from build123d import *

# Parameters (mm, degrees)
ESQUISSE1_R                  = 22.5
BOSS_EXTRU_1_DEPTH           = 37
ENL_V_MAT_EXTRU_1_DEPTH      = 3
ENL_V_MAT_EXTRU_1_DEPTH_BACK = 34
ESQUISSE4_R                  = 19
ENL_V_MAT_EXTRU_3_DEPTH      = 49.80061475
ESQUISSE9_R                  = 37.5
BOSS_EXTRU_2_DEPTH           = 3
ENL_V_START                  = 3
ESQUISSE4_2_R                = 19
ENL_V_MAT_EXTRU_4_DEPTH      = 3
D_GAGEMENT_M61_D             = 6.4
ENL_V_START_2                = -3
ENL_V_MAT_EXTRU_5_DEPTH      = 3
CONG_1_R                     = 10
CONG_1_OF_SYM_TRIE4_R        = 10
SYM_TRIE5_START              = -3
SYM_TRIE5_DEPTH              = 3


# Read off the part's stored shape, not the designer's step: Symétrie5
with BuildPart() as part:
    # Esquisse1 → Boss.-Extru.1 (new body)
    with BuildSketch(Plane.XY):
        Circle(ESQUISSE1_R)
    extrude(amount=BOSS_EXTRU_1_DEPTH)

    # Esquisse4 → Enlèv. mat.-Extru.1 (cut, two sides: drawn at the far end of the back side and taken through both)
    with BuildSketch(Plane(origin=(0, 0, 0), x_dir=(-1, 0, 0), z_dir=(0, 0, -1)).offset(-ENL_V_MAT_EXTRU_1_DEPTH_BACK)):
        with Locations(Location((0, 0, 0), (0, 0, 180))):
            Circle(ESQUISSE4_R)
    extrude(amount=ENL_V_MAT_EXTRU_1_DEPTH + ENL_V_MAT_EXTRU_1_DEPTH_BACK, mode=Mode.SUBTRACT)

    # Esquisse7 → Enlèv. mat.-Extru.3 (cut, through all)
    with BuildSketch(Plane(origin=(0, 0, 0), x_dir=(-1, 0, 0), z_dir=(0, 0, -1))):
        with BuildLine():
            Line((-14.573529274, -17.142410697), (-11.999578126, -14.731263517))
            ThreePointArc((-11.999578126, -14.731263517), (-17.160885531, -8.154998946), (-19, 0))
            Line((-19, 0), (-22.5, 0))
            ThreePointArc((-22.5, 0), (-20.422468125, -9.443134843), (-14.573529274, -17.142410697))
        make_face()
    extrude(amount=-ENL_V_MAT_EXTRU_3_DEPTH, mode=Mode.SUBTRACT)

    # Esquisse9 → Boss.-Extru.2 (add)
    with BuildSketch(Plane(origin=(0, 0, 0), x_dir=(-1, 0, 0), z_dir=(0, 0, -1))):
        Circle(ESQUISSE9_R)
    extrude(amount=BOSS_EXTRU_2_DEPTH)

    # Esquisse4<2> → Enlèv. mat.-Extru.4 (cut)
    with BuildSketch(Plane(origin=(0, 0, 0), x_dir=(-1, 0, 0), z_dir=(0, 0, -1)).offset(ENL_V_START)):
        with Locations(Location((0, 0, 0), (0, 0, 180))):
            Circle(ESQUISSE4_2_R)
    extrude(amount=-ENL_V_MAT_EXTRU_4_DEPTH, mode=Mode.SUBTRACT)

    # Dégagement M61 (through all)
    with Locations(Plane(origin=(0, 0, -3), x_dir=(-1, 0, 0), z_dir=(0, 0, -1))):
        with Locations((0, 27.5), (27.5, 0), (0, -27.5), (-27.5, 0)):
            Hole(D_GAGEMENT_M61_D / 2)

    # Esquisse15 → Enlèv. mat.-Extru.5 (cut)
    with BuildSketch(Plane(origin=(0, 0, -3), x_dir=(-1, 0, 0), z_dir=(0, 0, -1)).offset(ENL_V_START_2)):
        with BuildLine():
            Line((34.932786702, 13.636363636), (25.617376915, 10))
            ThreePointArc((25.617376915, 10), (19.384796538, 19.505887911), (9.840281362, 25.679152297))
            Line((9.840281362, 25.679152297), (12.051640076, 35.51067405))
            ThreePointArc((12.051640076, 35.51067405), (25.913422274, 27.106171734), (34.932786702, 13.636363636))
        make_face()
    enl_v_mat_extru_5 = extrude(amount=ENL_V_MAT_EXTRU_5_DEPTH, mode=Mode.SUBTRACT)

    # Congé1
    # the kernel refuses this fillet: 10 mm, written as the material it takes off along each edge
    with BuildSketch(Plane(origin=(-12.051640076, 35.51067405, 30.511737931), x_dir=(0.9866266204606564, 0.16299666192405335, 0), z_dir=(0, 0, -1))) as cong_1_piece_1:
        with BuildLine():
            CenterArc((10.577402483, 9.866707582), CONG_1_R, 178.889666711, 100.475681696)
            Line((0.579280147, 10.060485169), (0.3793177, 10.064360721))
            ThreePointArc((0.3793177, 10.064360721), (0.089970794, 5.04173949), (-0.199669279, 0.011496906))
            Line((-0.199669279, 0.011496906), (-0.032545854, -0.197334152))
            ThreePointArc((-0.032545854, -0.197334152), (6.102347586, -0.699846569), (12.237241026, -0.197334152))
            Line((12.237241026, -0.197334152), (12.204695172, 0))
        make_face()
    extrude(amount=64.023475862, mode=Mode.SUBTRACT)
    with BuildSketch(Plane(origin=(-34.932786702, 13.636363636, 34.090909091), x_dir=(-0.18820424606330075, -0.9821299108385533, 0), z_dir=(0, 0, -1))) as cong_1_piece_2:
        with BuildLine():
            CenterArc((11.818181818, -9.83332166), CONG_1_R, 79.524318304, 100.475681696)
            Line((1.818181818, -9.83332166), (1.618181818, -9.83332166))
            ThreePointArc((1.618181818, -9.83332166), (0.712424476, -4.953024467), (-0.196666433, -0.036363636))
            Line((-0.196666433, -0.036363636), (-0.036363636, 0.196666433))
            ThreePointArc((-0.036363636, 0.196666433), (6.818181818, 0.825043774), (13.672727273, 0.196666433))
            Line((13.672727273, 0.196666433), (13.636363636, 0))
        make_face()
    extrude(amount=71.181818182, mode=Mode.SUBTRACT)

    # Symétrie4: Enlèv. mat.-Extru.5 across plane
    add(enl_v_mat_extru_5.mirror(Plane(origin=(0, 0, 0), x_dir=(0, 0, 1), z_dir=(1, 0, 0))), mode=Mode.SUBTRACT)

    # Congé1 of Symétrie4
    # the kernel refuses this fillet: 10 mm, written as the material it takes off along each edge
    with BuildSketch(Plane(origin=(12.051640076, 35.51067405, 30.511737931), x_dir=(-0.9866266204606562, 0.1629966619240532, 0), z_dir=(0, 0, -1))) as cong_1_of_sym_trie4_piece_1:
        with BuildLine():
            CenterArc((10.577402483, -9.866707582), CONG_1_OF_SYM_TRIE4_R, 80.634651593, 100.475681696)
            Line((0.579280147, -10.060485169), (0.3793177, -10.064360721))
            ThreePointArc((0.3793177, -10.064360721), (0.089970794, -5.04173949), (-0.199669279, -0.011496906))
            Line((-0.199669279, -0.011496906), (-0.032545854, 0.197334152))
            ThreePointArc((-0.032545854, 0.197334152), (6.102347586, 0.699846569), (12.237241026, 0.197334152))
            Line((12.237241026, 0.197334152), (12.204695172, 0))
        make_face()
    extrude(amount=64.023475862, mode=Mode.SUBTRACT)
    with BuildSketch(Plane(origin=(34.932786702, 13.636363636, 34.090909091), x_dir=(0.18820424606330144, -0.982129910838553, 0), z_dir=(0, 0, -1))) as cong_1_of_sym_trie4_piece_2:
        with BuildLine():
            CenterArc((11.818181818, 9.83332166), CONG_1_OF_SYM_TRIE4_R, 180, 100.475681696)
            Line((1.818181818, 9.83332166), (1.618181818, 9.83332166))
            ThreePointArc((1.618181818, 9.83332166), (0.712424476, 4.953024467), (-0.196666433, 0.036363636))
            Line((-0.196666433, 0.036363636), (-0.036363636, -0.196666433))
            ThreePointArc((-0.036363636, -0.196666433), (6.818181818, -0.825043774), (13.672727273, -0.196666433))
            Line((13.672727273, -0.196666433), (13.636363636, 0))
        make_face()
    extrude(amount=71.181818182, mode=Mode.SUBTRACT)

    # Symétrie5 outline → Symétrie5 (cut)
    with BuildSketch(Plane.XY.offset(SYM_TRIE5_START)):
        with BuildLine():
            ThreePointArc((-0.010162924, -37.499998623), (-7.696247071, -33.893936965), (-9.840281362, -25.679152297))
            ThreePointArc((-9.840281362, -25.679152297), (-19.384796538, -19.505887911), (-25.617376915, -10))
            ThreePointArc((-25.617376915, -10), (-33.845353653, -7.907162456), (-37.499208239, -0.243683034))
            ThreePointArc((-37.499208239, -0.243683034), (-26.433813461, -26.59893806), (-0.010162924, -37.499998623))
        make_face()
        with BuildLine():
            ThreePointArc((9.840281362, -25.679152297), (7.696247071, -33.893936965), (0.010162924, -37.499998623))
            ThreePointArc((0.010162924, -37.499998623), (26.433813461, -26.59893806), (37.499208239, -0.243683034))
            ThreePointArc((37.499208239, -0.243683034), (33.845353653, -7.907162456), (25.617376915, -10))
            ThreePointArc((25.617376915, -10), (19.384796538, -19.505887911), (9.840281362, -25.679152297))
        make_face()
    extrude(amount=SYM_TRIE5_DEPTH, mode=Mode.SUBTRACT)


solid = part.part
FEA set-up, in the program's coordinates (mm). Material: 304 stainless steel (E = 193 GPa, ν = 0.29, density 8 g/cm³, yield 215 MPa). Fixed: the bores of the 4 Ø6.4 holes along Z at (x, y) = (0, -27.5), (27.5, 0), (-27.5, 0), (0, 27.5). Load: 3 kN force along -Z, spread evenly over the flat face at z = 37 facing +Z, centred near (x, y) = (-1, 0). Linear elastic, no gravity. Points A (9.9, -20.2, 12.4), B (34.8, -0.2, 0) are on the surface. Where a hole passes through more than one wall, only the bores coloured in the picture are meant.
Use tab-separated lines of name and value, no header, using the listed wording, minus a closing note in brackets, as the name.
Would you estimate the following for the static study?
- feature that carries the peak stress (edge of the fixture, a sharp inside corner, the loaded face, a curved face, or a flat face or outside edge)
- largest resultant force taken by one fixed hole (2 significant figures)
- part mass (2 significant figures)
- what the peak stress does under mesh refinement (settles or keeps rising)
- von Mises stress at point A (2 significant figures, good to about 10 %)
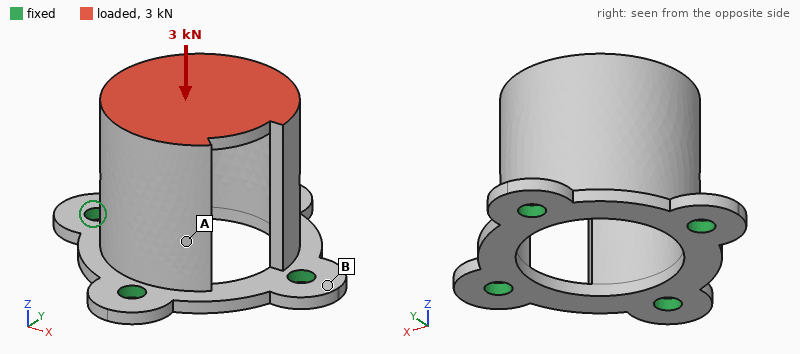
feature that carries the peak stress	edge of the fixture
largest resultant force taken by one fixed hole	970 N
part mass	190 g
what the peak stress does under mesh refinement	keeps rising
von Mises stress at point A	17 MPa
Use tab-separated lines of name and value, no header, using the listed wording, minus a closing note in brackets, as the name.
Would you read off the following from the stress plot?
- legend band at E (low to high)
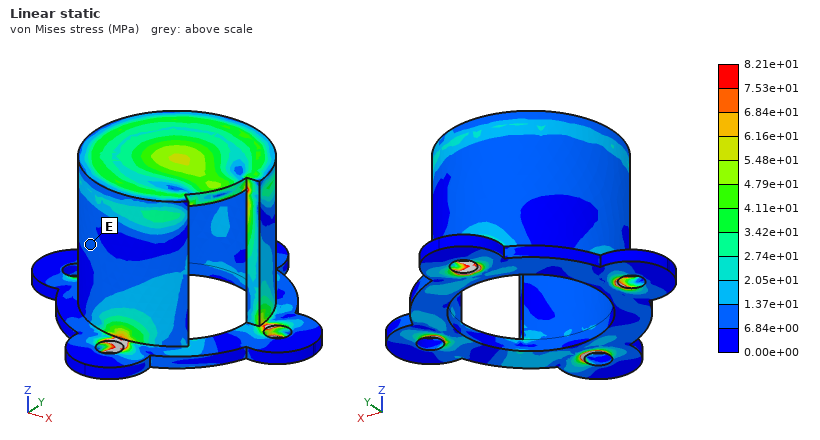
legend band at E	6.84e+00 to 1.37e+01 MPa
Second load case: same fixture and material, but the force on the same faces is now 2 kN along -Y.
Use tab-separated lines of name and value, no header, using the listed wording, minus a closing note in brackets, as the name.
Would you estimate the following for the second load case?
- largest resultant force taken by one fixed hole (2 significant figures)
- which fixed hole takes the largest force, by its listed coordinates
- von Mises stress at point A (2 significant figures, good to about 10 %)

largest resultant force taken by one fixed hole	2.5 kN
which fixed hole takes the largest force, by its listed coordinates	(0, 27.5)
von Mises stress at point A	22 MPa
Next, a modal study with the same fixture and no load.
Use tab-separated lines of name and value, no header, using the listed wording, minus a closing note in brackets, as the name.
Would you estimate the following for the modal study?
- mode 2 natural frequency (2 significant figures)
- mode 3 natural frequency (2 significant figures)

mode 2 natural frequency	5800 Hz
mode 3 natural frequency	9500 Hz
